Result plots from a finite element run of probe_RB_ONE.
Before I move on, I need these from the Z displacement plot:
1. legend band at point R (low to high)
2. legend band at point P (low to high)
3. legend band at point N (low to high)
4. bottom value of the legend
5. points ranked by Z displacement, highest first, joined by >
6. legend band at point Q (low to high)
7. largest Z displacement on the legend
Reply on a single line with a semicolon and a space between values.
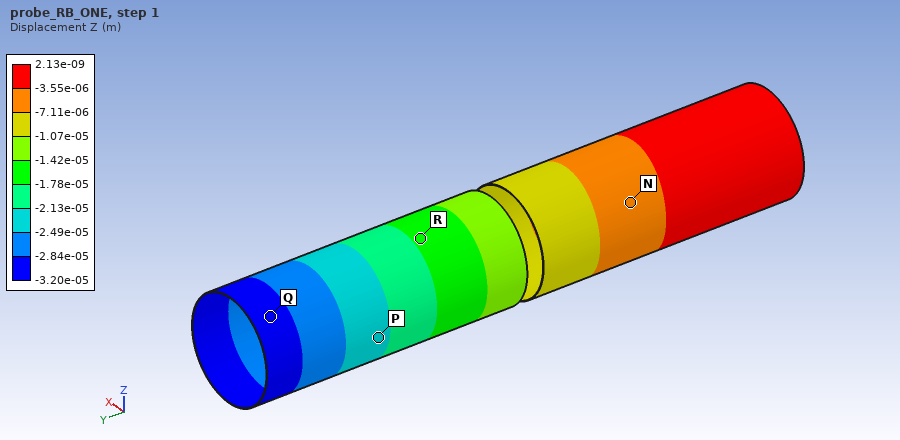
-1.78e-05 to -1.42e-05 m; -2.49e-05 to -2.13e-05 m; -7.11e-06 to -3.55e-06 m; -3.20e-05 m; N > R > P > Q; -3.20e-05 to -2.84e-05 m; 2.13e-09 m
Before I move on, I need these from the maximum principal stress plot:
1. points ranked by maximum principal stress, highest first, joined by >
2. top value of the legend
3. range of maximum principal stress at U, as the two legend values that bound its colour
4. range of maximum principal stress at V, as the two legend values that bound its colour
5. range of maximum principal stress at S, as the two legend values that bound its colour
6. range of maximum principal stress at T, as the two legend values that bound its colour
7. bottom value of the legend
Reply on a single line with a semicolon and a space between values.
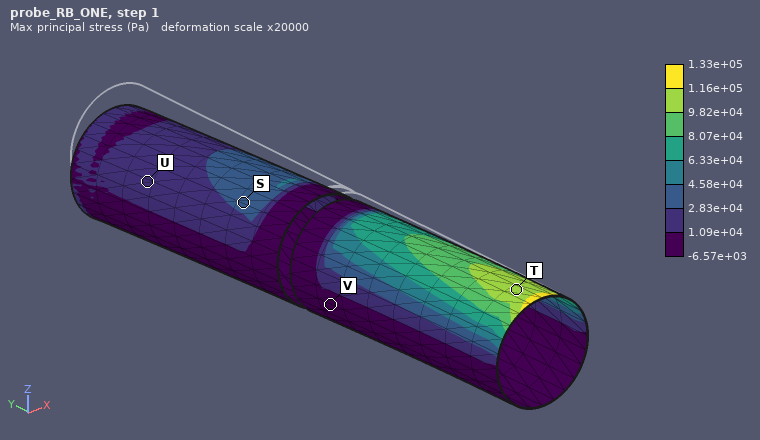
T > S > U > V; 1.33e+05 Pa; 1.09e+04 to 2.83e+04 Pa; -6.57e+03 to 1.09e+04 Pa; 2.83e+04 to 4.58e+04 Pa; 9.82e+04 to 1.16e+05 Pa; -6.57e+03 Pa
